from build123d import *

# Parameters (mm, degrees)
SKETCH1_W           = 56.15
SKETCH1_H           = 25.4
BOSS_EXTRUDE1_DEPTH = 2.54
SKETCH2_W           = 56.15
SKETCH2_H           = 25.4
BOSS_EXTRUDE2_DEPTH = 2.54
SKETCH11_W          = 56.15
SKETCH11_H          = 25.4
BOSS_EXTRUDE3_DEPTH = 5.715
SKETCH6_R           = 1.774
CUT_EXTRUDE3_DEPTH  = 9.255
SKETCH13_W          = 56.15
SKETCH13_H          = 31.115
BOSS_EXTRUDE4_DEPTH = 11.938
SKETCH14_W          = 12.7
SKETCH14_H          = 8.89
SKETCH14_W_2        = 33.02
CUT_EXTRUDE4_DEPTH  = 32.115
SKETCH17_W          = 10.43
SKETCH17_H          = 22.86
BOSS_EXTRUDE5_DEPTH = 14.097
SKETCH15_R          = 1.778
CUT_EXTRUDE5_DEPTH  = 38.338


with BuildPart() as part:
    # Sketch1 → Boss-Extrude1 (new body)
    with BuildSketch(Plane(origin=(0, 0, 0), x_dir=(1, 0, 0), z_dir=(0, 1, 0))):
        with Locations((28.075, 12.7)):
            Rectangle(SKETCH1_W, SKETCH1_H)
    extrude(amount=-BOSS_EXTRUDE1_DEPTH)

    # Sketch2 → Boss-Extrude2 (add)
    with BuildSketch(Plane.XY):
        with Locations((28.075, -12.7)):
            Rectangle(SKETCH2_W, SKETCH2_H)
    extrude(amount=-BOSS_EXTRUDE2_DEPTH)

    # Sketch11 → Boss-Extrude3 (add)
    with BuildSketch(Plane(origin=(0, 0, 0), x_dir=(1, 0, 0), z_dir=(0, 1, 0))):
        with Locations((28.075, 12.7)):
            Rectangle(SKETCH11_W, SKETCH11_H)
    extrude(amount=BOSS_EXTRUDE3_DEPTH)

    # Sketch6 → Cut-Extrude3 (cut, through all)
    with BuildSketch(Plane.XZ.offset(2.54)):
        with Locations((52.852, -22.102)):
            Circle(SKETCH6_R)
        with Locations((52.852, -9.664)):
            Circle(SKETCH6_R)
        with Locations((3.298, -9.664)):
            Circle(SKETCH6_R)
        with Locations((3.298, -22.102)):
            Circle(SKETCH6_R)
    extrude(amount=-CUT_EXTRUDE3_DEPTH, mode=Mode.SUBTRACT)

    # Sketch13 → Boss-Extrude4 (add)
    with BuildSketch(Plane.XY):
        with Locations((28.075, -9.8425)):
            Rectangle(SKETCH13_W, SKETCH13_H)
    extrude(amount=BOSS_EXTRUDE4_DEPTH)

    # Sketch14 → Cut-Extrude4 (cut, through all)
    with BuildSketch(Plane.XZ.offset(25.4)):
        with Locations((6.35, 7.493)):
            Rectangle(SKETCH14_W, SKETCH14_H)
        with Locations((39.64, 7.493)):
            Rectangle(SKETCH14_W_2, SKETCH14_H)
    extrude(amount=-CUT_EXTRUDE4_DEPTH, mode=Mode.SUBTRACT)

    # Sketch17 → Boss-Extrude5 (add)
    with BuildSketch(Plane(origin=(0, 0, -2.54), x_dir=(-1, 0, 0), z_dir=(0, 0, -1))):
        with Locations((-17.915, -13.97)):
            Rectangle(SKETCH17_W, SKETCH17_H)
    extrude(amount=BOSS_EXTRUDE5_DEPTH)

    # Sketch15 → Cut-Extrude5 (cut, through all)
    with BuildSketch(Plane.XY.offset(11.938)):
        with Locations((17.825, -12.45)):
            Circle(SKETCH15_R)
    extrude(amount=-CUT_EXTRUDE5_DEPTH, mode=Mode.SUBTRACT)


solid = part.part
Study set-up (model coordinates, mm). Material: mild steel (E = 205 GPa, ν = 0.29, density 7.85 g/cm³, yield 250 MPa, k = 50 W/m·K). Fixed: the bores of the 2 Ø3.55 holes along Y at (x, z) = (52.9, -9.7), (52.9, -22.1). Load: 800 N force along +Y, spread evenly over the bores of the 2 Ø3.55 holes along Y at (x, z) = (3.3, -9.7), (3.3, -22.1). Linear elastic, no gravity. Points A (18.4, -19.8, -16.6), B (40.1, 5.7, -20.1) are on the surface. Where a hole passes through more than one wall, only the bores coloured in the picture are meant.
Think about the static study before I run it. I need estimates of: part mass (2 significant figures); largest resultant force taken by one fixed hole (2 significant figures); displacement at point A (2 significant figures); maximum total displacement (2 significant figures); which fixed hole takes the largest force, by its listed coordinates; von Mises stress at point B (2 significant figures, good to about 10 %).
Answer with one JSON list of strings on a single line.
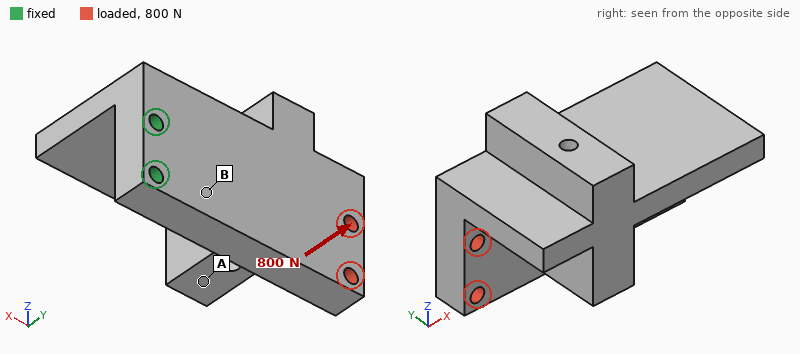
["200 g", "460 N", "66 µm", "99 µm", "(52.9, -9.7)", "59 MPa"]
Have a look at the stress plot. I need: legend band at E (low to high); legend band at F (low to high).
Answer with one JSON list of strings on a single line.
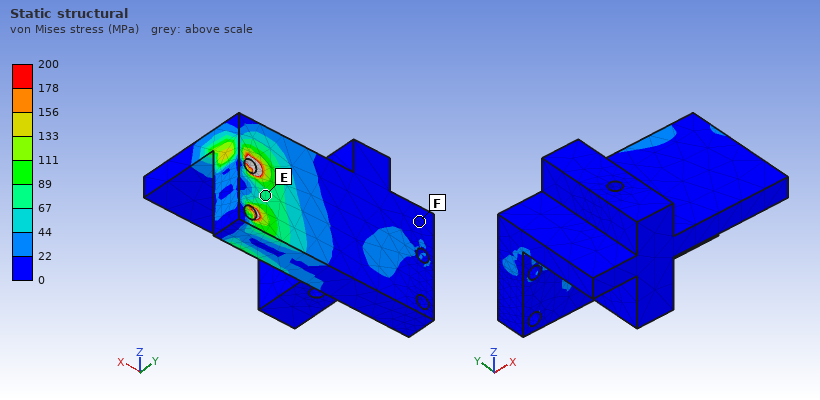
["67 to 89 MPa", "0 to 22 MPa"]
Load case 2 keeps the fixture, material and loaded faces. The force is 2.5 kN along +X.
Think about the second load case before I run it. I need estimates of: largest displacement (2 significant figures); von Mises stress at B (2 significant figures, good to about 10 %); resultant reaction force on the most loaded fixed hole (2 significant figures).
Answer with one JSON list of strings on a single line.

["6.6 µm", "17 MPa", "1.3 kN"]
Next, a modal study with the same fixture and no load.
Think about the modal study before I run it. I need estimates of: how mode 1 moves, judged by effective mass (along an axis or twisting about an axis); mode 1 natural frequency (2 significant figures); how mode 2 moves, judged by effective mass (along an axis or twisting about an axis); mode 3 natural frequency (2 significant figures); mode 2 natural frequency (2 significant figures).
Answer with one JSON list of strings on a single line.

["along Y", "1600 Hz", "along Z", "4700 Hz", "2900 Hz"]
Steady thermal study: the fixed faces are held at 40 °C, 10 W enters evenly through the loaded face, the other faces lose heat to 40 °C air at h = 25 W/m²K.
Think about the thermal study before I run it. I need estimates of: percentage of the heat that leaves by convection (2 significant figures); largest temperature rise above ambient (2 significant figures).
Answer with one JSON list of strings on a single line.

["31 %", "36 K"]
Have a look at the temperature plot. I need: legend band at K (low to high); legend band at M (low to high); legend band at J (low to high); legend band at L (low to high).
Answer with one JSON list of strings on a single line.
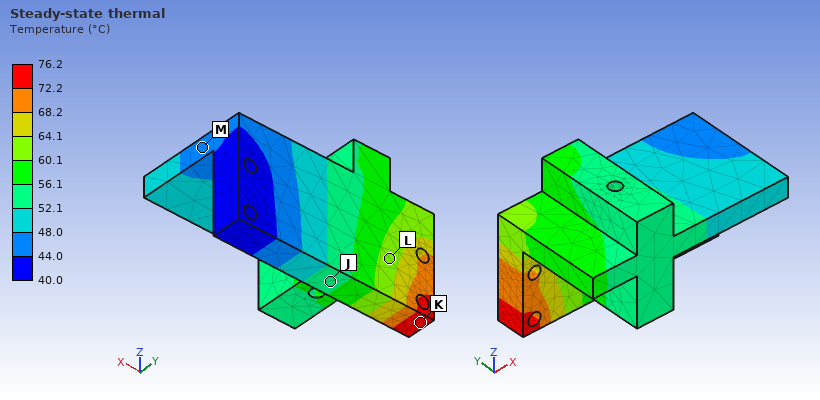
["72.2 to 76.2 °C", "44.0 to 48.0 °C", "52.1 to 56.1 °C", "60.1 to 64.1 °C"]
